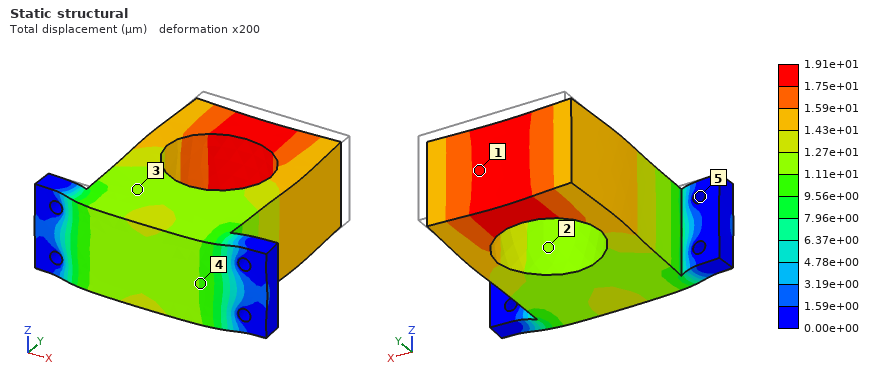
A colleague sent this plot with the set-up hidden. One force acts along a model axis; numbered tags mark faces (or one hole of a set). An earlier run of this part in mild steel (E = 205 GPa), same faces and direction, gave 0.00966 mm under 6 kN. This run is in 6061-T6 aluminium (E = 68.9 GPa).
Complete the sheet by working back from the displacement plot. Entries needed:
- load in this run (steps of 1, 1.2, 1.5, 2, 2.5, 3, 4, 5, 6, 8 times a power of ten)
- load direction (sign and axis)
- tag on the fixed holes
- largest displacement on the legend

4 kN
-Y
5
1.91e+01 µm
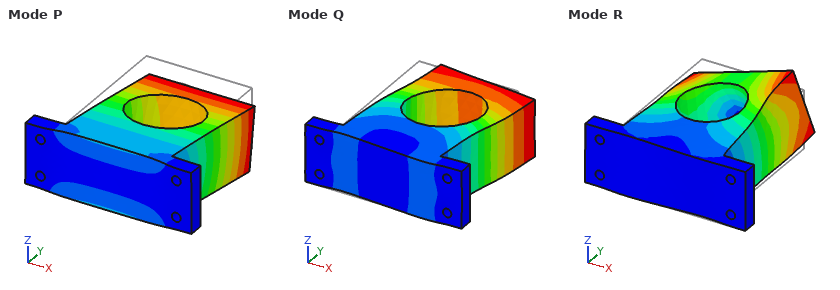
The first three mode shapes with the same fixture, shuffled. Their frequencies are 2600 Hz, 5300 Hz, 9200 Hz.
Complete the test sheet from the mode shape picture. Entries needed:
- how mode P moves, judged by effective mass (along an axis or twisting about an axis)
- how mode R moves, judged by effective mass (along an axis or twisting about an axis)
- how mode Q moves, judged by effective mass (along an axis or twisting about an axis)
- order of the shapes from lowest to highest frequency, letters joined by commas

along Z
twisting about Y
along X
P, Q, R
